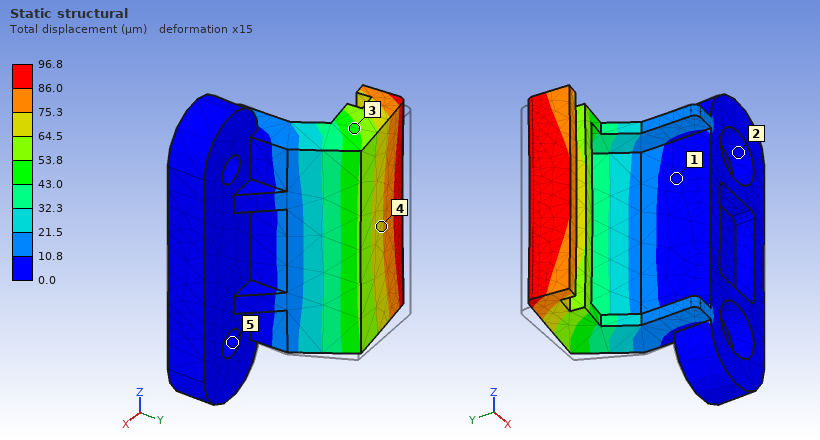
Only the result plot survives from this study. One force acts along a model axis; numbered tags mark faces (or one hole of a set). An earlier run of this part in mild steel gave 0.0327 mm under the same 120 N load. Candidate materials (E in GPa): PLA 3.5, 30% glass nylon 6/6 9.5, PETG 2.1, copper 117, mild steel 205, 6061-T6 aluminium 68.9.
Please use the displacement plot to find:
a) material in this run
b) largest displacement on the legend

6061-T6 aluminium
96.8 µm
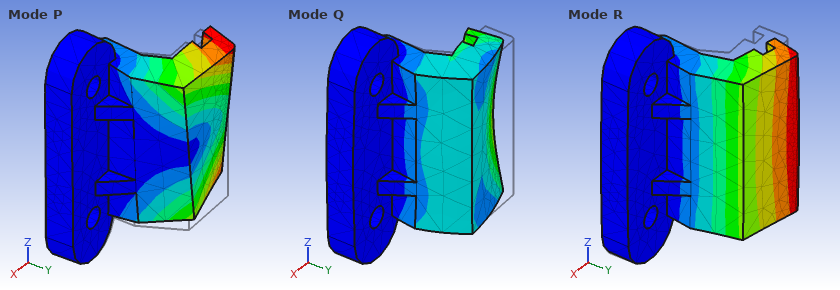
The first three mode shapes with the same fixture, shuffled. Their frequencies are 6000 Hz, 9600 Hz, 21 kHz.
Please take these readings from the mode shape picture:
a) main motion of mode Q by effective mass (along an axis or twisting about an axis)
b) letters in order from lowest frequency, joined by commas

along X
R, P, Q
